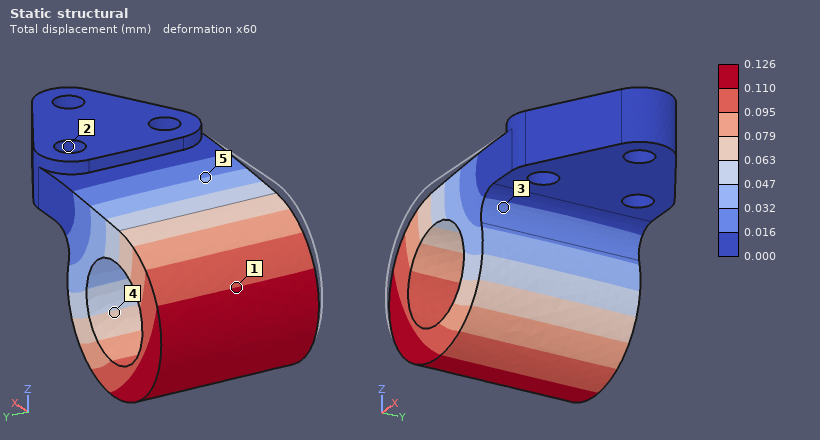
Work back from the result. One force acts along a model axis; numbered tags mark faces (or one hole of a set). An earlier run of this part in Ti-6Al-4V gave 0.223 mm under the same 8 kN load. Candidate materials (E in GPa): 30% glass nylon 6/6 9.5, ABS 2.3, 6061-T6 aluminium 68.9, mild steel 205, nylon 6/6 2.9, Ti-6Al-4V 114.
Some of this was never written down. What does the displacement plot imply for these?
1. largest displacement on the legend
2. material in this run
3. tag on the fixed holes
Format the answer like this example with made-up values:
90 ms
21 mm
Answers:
0.126 mm
mild steel
2
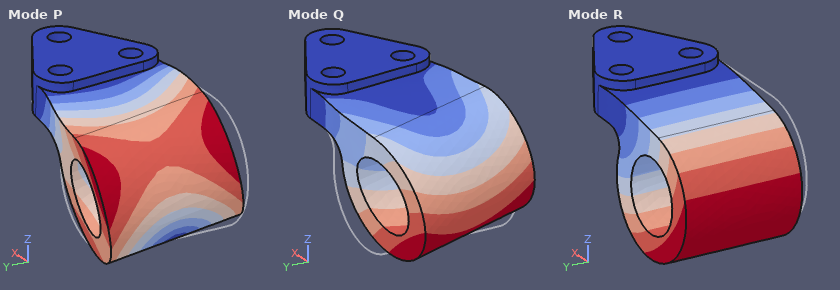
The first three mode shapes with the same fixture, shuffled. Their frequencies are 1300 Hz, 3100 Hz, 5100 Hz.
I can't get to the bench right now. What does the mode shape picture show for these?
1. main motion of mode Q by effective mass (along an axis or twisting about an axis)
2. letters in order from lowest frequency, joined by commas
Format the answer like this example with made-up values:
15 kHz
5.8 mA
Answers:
along Y
R, Q, P
